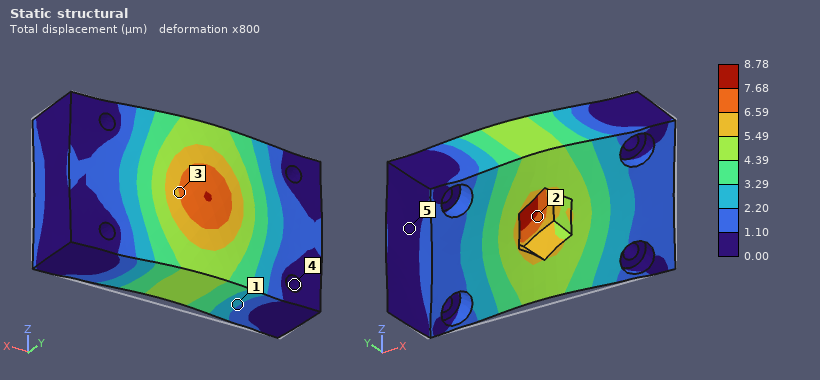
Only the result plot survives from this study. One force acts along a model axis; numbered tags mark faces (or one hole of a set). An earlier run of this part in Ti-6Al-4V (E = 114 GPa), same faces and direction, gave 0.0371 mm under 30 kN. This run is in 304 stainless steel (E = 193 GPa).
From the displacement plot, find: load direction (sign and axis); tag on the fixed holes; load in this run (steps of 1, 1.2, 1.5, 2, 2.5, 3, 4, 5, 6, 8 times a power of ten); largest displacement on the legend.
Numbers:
+Y
4
12 kN
8.78 µm
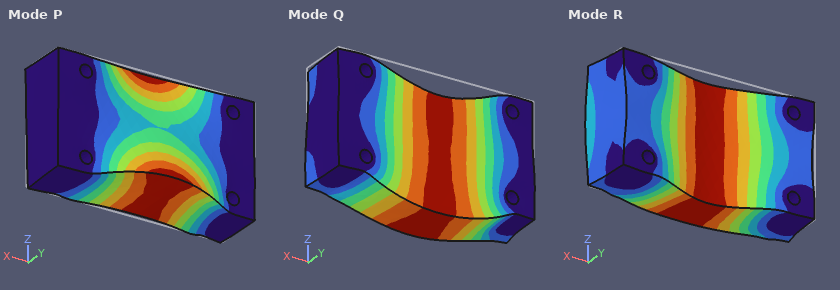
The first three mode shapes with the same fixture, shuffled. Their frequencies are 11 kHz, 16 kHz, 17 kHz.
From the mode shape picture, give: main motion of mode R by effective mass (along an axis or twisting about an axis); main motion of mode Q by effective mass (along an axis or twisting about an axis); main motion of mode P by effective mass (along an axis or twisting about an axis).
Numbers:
along Y
along Z
twisting about X
